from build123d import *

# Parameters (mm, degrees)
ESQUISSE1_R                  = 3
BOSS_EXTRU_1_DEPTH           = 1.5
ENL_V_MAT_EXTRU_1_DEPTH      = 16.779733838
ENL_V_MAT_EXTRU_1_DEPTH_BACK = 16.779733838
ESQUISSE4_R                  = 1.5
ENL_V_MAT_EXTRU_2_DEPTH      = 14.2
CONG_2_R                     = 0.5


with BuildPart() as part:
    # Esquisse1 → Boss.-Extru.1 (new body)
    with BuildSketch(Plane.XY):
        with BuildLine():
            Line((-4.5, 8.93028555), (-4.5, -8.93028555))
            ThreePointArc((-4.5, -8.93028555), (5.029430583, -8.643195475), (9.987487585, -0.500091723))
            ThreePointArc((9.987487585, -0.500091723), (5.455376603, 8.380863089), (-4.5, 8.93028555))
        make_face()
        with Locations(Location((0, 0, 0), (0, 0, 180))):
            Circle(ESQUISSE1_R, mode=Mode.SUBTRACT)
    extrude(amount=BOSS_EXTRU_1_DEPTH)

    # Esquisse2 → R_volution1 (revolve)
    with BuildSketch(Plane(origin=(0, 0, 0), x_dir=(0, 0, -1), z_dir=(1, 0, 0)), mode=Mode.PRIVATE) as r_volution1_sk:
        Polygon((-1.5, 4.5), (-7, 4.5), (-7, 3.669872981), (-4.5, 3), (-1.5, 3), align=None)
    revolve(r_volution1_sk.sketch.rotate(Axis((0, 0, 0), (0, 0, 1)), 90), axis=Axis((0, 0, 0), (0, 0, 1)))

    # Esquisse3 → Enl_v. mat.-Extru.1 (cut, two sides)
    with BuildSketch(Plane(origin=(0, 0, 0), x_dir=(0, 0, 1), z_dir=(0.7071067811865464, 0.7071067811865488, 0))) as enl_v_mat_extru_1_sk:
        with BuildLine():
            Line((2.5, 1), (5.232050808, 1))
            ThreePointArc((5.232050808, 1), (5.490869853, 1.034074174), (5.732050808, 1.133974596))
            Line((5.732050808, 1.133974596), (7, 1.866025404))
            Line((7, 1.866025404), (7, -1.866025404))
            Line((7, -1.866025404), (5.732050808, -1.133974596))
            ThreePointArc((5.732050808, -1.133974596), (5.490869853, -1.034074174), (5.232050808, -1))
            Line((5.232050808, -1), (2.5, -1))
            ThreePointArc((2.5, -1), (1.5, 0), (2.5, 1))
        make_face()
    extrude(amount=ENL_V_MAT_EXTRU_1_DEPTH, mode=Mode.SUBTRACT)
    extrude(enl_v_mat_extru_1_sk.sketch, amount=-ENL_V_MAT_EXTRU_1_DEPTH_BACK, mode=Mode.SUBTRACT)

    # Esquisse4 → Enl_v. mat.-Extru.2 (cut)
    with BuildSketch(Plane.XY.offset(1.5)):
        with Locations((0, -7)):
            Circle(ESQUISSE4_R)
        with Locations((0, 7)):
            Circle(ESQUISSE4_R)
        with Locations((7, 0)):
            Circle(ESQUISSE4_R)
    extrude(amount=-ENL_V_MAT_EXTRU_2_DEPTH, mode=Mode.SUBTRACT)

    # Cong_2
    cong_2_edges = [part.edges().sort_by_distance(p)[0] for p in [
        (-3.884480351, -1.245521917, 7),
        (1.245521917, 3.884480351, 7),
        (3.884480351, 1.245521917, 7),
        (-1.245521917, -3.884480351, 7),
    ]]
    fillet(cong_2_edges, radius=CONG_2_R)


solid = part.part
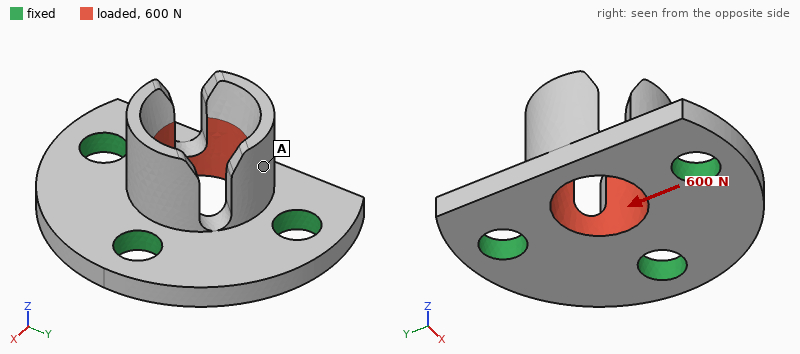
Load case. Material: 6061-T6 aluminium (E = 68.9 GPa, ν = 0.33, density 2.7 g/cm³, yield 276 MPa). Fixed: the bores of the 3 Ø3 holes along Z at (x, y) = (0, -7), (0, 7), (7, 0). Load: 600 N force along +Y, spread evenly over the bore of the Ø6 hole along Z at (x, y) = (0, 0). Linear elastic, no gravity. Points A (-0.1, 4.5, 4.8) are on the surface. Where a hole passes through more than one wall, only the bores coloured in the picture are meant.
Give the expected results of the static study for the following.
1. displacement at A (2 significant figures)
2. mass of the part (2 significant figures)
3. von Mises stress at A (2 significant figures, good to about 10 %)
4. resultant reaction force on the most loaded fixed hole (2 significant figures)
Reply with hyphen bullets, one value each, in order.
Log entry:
- 7.0 µm
- 1.2 g
- 16 MPa
- 260 N
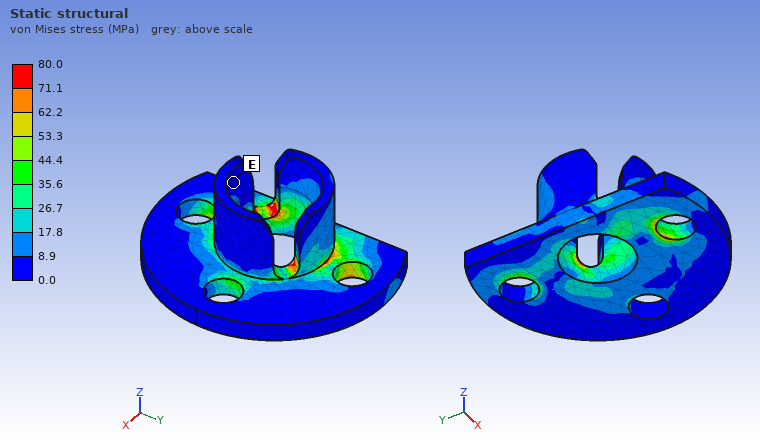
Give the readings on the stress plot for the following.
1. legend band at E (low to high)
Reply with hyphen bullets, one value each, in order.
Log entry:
- 0.0 to 8.9 MPa
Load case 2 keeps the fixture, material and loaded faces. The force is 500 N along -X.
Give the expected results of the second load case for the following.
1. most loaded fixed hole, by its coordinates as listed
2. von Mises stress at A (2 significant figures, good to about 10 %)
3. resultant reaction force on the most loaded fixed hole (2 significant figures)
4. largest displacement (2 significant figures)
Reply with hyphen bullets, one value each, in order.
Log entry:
- (7, 0)
- 11 MPa
- 210 N
- 23 µm
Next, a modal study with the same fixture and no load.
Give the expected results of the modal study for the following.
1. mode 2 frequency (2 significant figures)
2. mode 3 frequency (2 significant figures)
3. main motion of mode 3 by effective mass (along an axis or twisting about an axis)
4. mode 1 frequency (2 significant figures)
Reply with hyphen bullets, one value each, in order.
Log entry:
- 37 kHz
- 52 kHz
- along Y
- 29 kHz
